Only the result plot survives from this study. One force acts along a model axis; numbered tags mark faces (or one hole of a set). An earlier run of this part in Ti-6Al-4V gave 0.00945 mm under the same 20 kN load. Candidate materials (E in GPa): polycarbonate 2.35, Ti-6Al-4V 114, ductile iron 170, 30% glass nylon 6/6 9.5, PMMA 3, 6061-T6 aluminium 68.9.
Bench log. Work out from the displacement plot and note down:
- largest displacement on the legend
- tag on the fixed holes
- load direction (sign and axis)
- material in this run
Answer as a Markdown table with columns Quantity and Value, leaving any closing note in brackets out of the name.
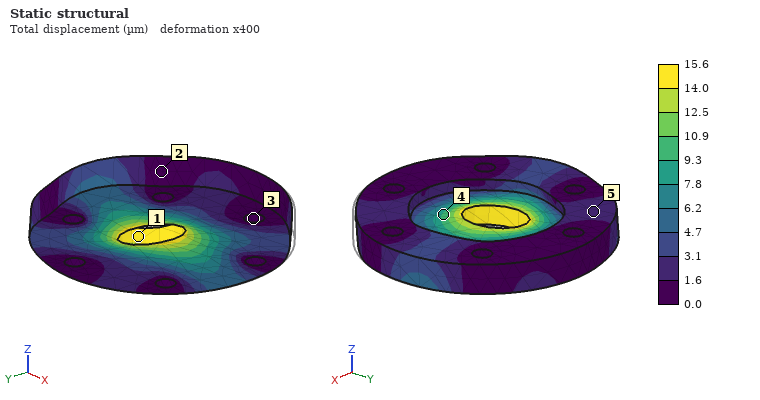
| Quantity | Value |
|---|---|
| largest displacement on the legend | 15.6 µm |
| tag on the fixed holes | 3 |
| load direction | -X |
| material in this run | 6061-T6 aluminium |
